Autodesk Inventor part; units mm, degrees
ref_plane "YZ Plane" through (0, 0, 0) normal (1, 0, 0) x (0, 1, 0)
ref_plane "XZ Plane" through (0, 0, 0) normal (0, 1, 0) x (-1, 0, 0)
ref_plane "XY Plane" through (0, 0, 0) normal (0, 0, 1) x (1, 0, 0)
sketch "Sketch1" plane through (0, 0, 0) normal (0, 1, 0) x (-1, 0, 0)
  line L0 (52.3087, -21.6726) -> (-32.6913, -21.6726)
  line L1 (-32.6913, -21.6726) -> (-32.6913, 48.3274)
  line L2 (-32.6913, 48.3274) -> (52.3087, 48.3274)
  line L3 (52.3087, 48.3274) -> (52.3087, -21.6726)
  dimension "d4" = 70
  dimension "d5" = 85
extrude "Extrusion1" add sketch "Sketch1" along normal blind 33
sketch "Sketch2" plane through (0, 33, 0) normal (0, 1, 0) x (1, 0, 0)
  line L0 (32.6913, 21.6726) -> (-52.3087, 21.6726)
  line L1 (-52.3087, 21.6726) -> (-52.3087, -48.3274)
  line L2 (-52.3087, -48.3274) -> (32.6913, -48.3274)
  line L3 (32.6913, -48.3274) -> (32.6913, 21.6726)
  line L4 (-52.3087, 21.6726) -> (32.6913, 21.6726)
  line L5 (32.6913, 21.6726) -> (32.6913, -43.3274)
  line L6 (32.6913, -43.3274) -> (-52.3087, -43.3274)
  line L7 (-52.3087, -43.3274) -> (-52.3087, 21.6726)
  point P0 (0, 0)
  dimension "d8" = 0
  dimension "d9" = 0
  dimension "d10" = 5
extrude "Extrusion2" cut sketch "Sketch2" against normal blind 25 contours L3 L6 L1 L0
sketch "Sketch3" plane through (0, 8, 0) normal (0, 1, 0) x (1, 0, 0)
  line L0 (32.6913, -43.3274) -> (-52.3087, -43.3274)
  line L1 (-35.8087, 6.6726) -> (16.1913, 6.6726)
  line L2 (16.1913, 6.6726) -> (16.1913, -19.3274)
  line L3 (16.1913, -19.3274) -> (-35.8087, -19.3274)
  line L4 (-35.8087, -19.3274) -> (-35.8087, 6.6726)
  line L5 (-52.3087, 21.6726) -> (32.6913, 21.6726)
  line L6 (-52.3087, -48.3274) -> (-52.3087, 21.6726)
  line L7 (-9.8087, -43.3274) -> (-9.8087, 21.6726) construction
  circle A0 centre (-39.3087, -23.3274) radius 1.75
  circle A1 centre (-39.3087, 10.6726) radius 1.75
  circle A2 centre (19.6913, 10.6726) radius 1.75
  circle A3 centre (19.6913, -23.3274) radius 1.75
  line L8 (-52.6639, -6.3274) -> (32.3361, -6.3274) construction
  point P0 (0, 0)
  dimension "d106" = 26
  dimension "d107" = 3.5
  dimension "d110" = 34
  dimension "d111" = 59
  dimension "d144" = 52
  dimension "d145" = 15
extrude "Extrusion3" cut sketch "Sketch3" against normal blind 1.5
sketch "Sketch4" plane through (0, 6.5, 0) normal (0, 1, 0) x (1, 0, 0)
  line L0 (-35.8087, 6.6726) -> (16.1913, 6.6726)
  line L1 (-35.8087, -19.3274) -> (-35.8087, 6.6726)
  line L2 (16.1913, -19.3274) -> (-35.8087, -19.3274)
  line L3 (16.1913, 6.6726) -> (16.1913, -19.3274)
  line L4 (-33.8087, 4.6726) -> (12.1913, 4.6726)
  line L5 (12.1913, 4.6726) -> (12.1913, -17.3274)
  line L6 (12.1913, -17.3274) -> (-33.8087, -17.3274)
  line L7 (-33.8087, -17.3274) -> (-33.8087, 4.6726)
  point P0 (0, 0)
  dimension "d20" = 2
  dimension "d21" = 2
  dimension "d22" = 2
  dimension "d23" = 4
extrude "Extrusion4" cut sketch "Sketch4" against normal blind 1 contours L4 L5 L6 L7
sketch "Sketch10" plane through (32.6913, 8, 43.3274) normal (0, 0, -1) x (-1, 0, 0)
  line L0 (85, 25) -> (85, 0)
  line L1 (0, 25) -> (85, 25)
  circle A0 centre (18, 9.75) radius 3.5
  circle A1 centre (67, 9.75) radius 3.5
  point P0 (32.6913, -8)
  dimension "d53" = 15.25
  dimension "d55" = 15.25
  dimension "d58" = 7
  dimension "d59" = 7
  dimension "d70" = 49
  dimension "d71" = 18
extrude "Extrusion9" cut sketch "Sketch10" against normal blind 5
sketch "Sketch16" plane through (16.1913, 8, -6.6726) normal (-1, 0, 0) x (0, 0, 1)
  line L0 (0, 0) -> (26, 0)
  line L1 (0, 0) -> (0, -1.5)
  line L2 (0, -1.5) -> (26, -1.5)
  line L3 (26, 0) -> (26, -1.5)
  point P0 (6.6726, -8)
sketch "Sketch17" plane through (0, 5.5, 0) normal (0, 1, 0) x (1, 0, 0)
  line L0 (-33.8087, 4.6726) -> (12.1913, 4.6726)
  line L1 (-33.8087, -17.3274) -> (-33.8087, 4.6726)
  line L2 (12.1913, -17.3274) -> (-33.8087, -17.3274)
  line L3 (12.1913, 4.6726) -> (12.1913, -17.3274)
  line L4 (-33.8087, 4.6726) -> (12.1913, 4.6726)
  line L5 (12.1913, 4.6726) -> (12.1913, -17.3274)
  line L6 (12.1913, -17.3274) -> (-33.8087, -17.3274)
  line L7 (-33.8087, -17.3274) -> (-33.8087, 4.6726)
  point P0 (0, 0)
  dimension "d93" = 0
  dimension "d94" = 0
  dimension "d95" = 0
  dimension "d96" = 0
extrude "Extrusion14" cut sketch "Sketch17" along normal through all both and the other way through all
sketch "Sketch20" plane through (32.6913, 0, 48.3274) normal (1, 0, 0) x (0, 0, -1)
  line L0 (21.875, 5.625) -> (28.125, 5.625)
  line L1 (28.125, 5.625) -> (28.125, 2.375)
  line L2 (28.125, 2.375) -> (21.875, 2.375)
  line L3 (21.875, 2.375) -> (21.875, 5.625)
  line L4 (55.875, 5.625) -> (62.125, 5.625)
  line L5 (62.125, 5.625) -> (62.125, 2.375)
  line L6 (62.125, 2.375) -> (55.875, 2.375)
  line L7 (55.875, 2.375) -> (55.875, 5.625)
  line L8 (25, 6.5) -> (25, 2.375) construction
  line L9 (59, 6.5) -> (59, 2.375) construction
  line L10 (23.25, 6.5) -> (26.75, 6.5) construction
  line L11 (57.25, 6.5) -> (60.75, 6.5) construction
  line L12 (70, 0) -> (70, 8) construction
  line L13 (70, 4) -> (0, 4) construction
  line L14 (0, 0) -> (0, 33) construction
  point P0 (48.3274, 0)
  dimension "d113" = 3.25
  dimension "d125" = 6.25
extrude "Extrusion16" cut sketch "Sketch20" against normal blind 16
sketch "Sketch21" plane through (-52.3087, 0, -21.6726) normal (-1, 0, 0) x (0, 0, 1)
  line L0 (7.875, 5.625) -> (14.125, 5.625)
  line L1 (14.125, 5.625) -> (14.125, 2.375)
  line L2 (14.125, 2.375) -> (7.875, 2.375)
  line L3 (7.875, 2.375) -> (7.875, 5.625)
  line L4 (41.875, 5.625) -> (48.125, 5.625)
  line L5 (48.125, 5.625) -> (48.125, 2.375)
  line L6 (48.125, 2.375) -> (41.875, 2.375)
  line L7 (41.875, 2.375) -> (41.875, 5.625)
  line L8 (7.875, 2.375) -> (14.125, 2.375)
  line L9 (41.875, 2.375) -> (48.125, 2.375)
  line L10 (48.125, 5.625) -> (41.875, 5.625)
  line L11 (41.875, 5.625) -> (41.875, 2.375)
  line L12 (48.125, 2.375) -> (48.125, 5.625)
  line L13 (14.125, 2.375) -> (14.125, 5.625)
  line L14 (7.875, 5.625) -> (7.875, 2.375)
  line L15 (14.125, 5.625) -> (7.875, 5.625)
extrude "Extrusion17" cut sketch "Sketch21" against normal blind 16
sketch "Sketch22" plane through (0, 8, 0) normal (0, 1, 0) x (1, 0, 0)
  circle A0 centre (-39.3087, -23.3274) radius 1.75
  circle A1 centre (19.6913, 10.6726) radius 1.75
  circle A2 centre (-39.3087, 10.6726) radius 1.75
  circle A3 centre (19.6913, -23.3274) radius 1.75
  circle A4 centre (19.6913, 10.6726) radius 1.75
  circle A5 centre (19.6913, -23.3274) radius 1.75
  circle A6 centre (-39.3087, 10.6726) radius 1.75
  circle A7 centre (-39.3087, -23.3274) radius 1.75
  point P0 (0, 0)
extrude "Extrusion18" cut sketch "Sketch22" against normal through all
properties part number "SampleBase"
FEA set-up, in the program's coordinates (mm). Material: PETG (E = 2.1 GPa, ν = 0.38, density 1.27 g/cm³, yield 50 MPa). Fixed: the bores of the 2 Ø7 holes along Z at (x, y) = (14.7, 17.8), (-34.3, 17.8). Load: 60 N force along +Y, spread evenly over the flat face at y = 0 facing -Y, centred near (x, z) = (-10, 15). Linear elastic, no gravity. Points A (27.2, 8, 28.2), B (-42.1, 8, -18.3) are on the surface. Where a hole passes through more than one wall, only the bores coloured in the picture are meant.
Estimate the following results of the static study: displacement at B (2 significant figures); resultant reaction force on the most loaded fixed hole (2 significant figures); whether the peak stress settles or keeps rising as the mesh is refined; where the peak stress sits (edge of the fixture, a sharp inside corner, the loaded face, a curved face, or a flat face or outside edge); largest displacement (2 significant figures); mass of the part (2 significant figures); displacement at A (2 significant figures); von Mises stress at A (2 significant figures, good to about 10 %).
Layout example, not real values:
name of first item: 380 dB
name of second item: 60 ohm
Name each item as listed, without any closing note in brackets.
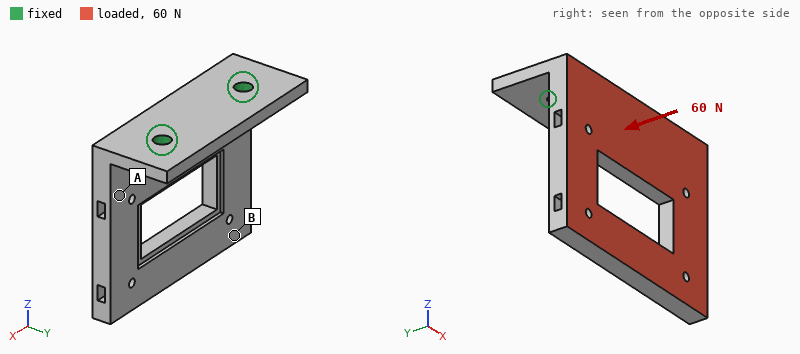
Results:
displacement at B: 1.1 mm
resultant reaction force on the most loaded fixed hole: 30 N
whether the peak stress settles or keeps rising as the mesh is refined: keeps rising
where the peak stress sits: edge of the fixture
largest displacement: 1.2 mm
mass of the part: 61 g
displacement at A: 0.23 mm
von Mises stress at A: 1.8 MPa
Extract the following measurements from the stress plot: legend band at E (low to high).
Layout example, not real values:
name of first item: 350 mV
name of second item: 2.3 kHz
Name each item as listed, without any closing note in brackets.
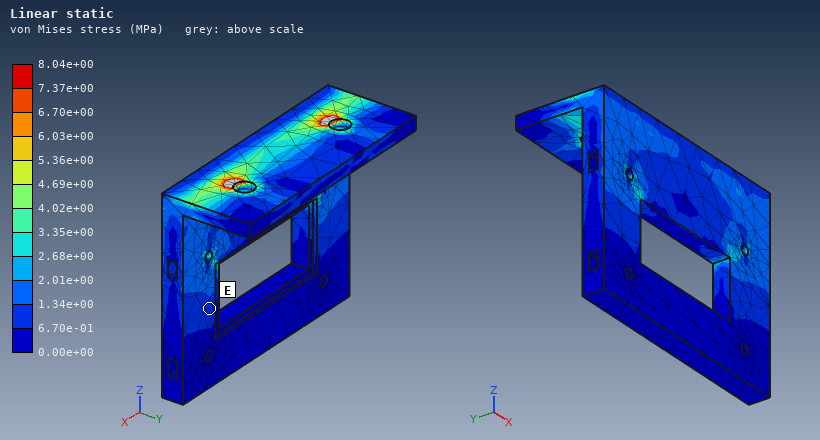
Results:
legend band at E: 6.70e-01 to 1.34e+00 MPa
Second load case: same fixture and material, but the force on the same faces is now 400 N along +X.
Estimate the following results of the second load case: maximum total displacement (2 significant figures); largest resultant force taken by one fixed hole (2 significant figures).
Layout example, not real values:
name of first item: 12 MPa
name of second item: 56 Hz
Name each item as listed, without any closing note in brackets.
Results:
maximum total displacement: 0.52 mm
largest resultant force taken by one fixed hole: 330 N
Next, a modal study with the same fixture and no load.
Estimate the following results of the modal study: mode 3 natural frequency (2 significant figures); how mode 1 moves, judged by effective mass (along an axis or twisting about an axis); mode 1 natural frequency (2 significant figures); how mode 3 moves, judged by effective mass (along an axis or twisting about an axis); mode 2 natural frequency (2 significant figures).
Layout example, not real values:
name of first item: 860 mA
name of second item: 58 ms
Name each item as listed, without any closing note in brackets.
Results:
mode 3 natural frequency: 780 Hz
how mode 1 moves, judged by effective mass: along Y
mode 1 natural frequency: 200 Hz
how mode 3 moves, judged by effective mass: along X
mode 2 natural frequency: 490 Hz
